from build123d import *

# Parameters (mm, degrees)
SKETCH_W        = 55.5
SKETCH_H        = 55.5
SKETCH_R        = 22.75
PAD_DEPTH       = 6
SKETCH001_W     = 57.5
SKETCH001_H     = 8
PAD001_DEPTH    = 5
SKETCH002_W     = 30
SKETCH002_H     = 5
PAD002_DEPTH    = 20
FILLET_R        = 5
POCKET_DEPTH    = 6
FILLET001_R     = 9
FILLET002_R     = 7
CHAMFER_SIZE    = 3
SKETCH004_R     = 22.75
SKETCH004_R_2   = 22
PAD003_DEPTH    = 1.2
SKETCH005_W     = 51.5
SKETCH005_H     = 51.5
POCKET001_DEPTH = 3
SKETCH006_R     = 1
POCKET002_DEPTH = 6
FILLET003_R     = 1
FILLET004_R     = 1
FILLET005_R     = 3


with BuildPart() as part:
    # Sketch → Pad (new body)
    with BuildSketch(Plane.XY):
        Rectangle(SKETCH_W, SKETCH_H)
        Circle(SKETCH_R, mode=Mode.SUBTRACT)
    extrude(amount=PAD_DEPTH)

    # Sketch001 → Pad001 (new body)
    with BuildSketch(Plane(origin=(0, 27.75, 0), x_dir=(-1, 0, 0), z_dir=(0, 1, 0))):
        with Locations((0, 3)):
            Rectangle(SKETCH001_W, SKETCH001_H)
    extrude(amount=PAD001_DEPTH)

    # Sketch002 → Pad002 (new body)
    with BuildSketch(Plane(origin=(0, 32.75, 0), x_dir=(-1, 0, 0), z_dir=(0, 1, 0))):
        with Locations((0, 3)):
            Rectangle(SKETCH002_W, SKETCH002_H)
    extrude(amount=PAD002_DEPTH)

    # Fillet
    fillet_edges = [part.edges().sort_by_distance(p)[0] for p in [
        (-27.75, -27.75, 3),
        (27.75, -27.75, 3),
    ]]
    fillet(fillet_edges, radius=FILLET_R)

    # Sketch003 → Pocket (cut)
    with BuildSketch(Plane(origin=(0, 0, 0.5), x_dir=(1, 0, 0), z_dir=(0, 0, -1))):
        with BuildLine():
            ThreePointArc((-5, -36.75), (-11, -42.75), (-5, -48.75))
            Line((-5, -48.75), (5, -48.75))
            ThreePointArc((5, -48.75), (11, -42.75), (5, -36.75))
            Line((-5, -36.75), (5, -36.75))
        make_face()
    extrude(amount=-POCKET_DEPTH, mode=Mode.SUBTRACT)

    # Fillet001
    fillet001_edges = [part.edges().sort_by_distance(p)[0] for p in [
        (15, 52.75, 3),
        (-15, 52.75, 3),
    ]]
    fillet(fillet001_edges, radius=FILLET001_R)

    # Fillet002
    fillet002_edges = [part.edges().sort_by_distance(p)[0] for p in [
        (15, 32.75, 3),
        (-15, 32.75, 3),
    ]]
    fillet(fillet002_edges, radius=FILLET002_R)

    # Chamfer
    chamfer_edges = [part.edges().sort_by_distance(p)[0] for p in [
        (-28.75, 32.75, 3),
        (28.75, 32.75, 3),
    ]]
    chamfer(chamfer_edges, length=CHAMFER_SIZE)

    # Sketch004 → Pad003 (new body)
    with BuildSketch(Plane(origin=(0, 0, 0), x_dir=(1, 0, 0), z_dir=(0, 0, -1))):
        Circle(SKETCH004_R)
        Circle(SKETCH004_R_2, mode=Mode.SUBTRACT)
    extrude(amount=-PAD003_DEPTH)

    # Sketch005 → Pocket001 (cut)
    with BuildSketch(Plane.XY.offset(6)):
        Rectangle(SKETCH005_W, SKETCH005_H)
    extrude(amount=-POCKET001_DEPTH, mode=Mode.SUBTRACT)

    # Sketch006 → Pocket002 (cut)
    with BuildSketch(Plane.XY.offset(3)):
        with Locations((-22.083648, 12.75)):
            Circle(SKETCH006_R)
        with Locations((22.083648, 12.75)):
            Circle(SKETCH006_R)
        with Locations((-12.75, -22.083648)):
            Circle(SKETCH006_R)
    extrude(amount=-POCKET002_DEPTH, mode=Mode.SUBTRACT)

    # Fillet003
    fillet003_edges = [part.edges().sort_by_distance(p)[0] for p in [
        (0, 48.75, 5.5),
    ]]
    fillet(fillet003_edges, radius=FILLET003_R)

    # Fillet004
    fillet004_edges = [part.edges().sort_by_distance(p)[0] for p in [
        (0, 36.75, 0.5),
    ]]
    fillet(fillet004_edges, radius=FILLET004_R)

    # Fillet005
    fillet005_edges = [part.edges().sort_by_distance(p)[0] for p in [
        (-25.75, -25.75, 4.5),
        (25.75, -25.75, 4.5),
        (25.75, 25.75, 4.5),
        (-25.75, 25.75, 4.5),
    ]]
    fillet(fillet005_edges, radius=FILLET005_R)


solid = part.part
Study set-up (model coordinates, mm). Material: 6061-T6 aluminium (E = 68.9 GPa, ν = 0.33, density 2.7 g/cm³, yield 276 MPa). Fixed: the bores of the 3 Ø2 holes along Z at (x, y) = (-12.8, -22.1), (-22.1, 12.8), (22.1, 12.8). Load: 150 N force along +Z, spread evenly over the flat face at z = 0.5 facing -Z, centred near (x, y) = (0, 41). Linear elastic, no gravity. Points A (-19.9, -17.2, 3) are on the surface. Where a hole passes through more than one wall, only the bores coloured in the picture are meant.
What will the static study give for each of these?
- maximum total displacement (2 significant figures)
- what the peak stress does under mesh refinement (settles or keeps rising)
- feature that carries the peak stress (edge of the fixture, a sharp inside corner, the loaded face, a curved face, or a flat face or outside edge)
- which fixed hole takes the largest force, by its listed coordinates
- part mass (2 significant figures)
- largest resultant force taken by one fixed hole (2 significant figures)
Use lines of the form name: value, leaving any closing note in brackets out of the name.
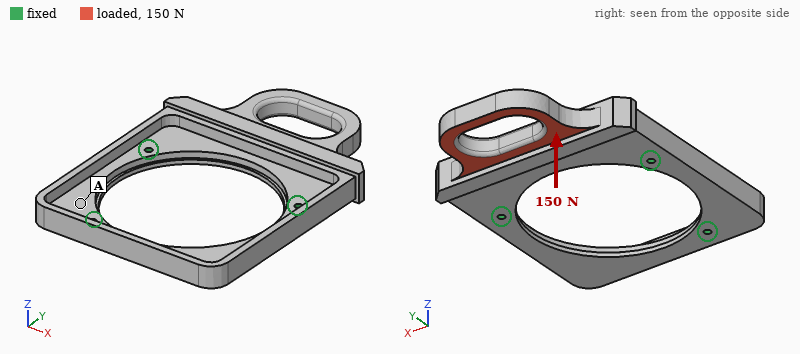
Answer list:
maximum total displacement: 0.26 mm
what the peak stress does under mesh refinement: keeps rising
feature that carries the peak stress: edge of the fixture
which fixed hole takes the largest force, by its listed coordinates: (-22.1, 12.8)
part mass: 26 g
largest resultant force taken by one fixed hole: 110 N
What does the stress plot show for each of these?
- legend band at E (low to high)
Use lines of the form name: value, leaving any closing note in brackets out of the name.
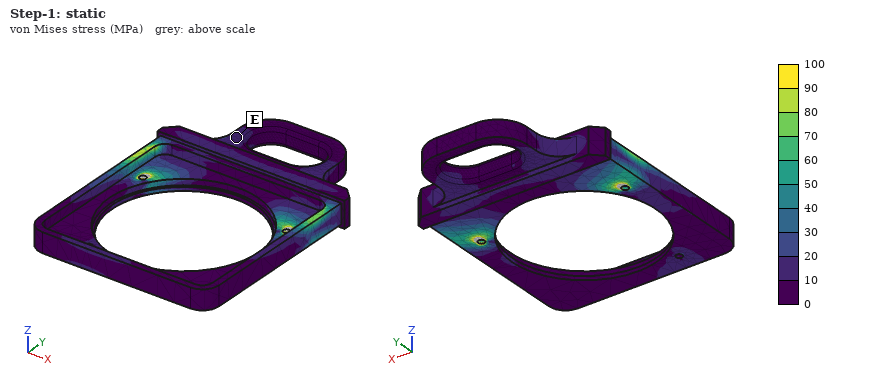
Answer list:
legend band at E: 10 to 20 MPa
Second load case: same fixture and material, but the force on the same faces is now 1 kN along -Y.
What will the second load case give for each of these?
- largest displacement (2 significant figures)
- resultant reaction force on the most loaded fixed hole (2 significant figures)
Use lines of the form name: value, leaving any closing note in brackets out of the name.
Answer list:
largest displacement: 0.12 mm
resultant reaction force on the most loaded fixed hole: 550 N
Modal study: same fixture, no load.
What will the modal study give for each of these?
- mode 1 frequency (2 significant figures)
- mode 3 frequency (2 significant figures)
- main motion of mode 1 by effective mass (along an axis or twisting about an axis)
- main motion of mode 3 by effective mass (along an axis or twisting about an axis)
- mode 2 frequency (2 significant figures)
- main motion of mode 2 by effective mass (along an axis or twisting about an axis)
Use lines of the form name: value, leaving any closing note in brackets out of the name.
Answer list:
mode 1 frequency: 1700 Hz
mode 3 frequency: 6100 Hz
main motion of mode 1 by effective mass: along Z
main motion of mode 3 by effective mass: twisting about Y
mode 2 frequency: 2600 Hz
main motion of mode 2 by effective mass: along Z
